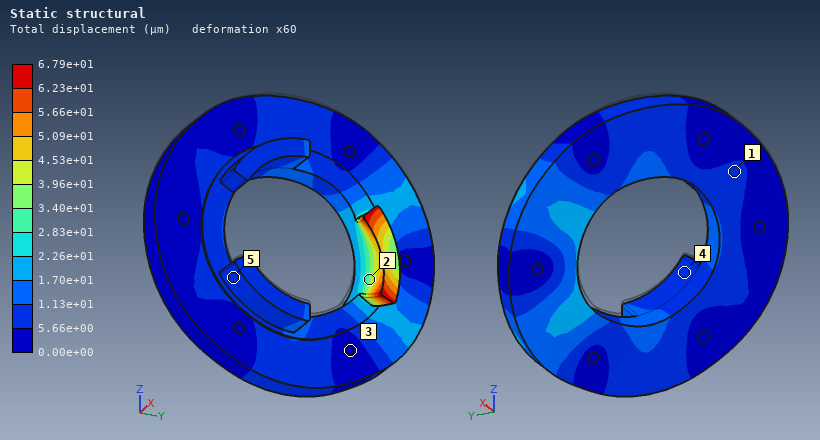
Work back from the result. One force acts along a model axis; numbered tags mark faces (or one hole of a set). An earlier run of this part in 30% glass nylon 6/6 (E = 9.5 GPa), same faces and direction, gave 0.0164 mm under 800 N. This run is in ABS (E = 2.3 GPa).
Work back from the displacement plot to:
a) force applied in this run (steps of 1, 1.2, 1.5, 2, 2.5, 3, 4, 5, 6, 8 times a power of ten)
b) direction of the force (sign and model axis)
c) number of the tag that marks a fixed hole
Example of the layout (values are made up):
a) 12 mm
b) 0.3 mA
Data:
a) 800 N
b) -Z
c) 3
